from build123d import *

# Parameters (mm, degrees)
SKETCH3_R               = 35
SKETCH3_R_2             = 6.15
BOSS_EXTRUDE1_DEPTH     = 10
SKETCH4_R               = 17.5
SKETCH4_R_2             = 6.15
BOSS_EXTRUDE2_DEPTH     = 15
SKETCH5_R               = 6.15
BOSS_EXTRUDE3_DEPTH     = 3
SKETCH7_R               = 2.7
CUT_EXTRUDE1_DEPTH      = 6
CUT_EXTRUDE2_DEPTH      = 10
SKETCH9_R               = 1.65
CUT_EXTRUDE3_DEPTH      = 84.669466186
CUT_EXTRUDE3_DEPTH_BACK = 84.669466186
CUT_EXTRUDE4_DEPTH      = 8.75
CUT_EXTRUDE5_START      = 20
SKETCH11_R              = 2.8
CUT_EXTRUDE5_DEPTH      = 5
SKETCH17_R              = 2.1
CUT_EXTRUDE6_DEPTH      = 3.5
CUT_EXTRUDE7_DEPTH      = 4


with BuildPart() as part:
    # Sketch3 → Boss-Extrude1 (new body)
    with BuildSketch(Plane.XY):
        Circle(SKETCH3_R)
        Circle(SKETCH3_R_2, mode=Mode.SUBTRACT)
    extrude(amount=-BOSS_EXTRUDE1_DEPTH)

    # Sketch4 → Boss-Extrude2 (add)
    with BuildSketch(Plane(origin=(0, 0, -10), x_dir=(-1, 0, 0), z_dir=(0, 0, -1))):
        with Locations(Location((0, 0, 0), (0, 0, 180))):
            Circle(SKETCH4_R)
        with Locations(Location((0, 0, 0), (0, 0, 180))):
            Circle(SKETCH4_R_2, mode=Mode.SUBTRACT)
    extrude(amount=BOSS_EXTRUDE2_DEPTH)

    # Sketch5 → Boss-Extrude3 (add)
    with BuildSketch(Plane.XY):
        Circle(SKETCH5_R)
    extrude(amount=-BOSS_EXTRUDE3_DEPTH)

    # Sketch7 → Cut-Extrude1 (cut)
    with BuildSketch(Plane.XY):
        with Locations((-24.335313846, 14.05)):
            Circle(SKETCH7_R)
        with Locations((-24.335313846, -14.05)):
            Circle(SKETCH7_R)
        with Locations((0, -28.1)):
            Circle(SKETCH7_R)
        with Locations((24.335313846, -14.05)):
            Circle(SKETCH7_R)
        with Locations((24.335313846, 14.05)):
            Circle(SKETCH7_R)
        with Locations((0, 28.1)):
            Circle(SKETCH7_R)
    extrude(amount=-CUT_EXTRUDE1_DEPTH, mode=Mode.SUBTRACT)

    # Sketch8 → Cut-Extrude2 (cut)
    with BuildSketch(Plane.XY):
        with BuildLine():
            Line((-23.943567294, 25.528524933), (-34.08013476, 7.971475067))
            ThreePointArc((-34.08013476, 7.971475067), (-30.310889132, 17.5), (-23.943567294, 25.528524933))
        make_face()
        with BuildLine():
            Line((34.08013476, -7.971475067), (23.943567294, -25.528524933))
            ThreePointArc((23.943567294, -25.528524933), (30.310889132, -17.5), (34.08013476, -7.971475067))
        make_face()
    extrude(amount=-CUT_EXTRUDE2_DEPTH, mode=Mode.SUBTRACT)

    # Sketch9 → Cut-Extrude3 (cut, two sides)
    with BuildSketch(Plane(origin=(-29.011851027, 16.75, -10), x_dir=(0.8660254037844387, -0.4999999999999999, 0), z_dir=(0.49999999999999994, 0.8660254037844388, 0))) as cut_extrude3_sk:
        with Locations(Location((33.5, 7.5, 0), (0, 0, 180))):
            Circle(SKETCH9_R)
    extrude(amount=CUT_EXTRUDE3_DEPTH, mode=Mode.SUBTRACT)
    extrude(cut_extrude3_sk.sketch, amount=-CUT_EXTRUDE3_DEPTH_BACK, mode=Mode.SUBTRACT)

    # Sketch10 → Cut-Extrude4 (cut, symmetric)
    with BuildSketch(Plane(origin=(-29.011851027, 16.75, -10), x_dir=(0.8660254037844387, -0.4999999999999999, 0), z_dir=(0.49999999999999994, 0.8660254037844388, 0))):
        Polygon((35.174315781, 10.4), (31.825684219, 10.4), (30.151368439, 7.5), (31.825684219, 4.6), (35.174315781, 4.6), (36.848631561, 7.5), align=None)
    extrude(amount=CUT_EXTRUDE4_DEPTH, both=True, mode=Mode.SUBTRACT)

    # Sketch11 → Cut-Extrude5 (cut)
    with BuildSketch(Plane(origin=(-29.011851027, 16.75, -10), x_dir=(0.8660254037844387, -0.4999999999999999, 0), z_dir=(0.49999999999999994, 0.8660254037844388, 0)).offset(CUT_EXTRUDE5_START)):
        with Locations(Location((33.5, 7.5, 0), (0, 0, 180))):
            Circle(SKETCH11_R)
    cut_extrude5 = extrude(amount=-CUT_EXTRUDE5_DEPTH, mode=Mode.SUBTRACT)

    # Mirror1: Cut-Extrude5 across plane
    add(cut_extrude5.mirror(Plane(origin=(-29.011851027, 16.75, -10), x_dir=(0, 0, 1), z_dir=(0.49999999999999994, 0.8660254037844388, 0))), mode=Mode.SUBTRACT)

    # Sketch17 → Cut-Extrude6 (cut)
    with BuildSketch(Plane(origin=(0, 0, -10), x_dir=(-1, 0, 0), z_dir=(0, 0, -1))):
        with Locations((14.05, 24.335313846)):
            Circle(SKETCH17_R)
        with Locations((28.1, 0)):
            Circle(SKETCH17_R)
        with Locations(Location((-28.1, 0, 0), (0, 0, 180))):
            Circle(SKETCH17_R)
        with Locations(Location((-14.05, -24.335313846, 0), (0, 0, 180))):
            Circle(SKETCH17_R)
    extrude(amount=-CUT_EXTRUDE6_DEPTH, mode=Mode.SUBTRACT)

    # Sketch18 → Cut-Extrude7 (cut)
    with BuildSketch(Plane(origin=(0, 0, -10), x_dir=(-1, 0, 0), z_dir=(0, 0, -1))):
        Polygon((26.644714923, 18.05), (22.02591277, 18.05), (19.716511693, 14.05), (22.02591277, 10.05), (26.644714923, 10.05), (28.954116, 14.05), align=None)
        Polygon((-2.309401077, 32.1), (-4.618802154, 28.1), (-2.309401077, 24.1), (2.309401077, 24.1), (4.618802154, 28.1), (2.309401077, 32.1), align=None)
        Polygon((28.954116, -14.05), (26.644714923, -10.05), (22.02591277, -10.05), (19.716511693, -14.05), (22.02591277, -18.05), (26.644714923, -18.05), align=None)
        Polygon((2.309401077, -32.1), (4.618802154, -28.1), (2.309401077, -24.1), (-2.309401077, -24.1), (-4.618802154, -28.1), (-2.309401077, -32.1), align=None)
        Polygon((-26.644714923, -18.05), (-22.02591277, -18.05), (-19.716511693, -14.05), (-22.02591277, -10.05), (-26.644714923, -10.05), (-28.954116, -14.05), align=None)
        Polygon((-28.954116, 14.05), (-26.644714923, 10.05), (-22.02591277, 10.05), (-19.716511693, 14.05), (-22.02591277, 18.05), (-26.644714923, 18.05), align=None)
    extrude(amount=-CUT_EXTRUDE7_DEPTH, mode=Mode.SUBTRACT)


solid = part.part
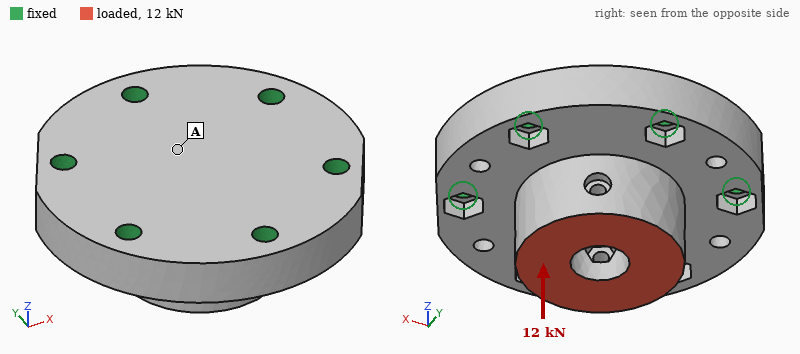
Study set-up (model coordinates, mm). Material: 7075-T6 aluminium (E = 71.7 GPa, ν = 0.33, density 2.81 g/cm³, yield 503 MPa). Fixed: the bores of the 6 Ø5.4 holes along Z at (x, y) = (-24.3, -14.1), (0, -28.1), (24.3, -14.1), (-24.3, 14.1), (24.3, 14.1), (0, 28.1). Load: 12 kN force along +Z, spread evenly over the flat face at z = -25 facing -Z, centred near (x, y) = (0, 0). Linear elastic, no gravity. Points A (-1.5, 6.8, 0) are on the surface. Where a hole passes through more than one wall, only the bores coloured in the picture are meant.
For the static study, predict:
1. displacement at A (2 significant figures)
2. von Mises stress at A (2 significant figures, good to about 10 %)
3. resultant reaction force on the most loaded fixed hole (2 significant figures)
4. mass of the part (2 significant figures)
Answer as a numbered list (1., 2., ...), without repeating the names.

1. 14 µm
2. 17 MPa
3. 2.4 kN
4. 130 g
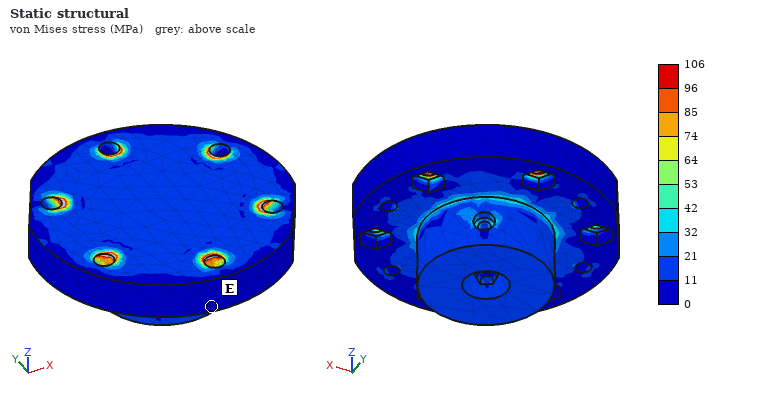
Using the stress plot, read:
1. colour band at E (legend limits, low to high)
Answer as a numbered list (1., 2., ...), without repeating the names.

1. 0 to 11 MPa
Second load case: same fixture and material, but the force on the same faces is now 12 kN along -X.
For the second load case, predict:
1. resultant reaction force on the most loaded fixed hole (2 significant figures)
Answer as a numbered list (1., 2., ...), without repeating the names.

1. 4.0 kN
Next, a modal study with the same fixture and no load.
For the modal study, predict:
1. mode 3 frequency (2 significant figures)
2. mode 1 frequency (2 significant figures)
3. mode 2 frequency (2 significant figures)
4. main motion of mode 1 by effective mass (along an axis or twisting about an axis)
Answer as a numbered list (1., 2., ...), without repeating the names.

1. 21 kHz
2. 18 kHz
3. 21 kHz
4. along Z
